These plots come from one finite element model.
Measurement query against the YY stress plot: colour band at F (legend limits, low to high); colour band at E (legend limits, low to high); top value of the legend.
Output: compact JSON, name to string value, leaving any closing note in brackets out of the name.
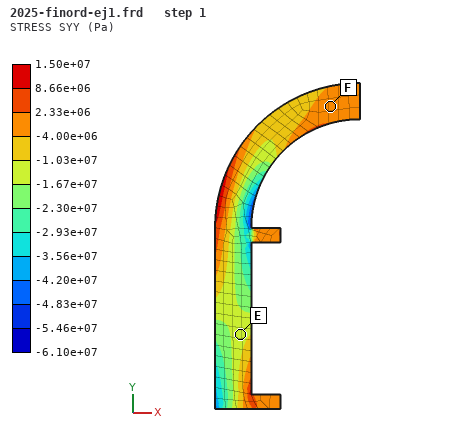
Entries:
{"colour band at F": "-4.00e+06 to 2.33e+06 Pa", "colour band at E": "-1.67e+07 to -1.03e+07 Pa", "top value of the legend": "1.50e+07 Pa"}
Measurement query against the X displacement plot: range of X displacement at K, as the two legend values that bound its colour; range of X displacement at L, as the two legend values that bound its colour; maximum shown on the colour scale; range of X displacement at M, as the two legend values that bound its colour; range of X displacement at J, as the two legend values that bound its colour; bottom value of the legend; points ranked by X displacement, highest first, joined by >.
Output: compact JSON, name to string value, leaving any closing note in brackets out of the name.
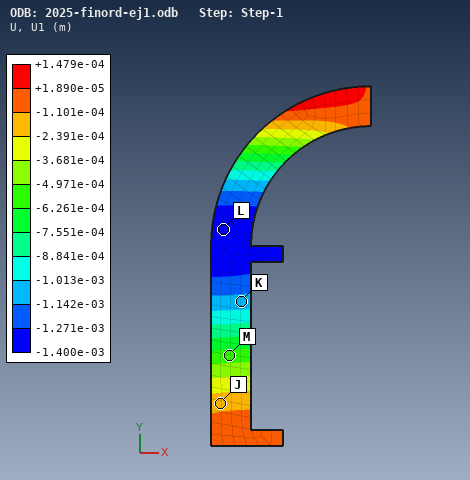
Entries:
{"range of X displacement at K, as the two legend values that bound its colour": "-1.142e-03 to -1.013e-03 m", "range of X displacement at L, as the two legend values that bound its colour": "-1.400e-03 to -1.271e-03 m", "maximum shown on the colour scale": "+1.479e-04 m", "range of X displacement at M, as the two legend values that bound its colour": "-6.261e-04 to -4.971e-04 m", "range of X displacement at J, as the two legend values that bound its colour": "-2.391e-04 to -1.101e-04 m", "bottom value of the legend": "-1.400e-03 m", "points ranked by X displacement, highest first, joined by >": "J > M > K > L"}
